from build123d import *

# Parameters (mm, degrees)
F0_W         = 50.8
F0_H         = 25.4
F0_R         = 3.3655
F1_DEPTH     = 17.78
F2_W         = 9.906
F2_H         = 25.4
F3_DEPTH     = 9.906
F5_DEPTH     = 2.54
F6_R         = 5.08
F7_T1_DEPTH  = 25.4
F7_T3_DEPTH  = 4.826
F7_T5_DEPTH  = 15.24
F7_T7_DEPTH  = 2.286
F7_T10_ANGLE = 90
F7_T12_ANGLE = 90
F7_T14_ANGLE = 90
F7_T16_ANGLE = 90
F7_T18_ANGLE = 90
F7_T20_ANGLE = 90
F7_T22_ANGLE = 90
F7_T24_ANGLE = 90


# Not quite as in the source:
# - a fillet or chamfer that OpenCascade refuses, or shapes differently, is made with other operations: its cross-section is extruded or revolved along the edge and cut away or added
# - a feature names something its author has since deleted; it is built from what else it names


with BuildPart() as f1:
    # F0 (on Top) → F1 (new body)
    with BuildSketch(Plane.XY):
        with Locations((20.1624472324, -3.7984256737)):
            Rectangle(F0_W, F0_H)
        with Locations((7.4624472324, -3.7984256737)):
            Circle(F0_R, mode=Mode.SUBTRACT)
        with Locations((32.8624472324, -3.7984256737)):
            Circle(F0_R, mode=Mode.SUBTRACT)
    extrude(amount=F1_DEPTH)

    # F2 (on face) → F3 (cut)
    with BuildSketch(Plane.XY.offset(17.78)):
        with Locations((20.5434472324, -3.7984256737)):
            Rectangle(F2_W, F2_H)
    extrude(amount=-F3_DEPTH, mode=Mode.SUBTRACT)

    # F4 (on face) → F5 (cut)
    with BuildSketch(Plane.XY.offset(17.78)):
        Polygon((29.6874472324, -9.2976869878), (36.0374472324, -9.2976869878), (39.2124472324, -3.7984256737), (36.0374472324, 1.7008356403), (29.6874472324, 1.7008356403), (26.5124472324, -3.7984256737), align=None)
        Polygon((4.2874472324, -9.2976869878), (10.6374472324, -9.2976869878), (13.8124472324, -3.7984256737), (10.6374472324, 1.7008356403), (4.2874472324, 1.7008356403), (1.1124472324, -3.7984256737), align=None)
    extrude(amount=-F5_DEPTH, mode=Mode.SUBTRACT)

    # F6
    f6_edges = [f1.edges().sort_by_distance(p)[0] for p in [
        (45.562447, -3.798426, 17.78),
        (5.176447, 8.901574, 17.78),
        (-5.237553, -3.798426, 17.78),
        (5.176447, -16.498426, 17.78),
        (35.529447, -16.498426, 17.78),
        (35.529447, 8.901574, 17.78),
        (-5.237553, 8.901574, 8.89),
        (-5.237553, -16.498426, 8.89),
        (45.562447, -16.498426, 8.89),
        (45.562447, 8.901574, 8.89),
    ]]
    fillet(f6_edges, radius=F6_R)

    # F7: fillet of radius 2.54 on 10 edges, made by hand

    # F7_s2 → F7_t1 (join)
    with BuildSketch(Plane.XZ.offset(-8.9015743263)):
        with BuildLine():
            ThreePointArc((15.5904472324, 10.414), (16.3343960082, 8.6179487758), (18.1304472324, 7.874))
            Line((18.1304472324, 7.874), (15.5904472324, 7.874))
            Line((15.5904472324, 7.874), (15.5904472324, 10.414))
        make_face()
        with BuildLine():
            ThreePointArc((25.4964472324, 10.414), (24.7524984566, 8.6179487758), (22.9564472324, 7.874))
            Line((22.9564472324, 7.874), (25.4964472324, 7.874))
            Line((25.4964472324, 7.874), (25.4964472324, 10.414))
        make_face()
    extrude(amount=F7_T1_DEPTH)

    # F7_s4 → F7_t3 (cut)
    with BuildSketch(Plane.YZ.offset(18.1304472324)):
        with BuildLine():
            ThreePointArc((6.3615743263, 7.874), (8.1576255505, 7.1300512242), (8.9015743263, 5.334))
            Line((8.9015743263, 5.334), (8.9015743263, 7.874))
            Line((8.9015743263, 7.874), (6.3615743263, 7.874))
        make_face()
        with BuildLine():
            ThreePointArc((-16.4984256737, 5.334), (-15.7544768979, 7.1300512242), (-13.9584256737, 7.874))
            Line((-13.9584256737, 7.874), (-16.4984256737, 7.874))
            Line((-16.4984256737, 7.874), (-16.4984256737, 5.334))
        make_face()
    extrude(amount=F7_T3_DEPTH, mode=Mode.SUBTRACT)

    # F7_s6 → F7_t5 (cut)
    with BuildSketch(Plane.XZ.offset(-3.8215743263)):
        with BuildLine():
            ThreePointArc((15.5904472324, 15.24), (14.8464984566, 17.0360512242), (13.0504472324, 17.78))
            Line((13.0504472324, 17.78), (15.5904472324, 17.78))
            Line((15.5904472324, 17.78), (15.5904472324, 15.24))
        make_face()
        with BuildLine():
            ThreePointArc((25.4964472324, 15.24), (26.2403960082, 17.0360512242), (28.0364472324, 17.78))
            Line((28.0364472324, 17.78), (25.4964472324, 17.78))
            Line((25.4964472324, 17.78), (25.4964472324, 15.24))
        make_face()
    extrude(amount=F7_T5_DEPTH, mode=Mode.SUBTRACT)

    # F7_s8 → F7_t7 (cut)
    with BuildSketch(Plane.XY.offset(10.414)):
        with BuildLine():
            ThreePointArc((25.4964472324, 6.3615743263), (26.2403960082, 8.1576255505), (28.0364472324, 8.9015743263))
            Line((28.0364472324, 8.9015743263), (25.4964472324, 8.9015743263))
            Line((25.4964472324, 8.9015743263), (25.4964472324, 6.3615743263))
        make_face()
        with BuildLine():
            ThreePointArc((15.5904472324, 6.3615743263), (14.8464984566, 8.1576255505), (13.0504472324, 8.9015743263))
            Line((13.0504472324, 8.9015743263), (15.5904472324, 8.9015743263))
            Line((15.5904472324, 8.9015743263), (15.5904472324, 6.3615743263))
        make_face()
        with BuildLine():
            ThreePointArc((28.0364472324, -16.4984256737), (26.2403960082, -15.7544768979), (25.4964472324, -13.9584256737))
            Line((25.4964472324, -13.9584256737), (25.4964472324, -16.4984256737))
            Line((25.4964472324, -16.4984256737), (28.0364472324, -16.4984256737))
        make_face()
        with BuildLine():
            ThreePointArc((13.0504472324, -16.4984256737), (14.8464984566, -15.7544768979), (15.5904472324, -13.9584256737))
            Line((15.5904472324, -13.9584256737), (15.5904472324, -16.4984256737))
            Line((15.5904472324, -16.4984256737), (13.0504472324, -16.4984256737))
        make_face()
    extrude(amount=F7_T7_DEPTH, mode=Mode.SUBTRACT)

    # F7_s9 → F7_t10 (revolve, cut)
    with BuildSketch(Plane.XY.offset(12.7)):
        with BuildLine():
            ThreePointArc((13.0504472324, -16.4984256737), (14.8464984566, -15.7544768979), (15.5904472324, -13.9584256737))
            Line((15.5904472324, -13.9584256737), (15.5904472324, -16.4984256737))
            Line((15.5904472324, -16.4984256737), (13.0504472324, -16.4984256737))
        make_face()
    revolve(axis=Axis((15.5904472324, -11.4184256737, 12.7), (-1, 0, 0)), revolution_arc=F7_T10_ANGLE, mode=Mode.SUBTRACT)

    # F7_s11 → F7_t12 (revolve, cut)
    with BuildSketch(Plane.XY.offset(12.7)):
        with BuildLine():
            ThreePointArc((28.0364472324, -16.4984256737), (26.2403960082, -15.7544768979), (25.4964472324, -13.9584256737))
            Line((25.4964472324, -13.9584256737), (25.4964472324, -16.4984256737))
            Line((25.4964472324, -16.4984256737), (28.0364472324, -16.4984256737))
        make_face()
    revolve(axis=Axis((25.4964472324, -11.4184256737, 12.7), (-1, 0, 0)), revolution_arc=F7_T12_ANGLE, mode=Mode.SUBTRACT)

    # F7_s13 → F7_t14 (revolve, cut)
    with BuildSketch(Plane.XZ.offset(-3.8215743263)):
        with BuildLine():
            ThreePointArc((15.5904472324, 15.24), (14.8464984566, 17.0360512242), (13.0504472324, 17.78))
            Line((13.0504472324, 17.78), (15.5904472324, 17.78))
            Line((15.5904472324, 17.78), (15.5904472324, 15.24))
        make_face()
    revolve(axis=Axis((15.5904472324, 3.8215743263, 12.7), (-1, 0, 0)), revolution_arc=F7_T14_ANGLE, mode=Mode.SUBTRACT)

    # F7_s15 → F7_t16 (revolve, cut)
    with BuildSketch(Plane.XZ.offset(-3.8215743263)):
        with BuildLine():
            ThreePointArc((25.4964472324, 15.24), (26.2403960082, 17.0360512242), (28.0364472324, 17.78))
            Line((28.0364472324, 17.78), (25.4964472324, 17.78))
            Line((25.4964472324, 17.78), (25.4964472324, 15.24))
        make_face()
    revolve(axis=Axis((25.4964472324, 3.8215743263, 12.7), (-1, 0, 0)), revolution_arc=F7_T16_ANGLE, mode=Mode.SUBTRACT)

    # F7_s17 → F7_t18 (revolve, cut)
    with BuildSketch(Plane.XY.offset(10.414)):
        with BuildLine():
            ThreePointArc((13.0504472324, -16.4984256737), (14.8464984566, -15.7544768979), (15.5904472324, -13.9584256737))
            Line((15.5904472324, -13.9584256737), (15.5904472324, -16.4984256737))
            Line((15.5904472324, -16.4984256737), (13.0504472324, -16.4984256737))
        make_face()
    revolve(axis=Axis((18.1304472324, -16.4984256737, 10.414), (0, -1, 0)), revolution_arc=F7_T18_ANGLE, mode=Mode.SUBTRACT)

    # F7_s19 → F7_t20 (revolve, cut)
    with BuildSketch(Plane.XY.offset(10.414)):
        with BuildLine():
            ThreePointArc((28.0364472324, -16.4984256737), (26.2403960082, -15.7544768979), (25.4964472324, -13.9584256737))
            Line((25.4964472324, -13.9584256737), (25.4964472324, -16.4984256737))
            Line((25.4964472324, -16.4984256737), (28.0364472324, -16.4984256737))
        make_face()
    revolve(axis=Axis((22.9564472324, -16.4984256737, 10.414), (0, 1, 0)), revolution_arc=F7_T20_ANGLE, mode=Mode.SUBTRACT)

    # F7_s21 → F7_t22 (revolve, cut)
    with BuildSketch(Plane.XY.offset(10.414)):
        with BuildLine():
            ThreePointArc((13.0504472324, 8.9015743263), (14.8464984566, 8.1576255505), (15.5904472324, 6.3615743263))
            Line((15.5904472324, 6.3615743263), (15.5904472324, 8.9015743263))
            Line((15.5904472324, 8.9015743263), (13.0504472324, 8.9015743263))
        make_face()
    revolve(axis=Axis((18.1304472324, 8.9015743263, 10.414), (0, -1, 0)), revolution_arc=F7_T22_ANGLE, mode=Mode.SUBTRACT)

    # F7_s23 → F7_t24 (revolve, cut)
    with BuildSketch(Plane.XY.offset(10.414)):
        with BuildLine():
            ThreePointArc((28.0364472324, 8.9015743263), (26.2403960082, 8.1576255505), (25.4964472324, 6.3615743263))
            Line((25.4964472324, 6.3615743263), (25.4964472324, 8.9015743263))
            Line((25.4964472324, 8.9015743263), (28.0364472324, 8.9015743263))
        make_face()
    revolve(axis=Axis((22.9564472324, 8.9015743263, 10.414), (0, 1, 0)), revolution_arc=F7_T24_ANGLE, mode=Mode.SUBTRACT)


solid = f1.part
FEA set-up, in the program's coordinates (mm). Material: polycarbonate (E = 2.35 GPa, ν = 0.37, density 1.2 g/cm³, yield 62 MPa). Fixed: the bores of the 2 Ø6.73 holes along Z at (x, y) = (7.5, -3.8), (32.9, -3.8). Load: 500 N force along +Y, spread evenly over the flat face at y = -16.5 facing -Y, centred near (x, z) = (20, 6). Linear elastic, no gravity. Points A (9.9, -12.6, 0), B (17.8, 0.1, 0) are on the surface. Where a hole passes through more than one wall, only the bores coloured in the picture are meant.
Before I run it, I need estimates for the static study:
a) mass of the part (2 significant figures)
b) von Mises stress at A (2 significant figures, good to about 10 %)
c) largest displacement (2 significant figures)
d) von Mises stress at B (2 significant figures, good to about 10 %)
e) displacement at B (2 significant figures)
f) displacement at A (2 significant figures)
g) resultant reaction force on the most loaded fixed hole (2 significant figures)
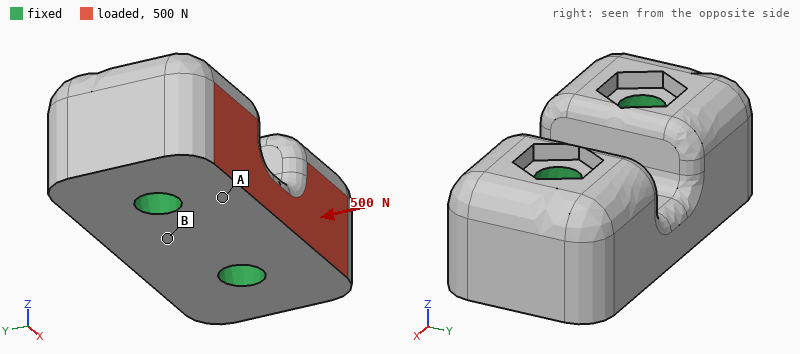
21 g
1.4 MPa
10 µm
0.41 MPa
2.9 µm
5.5 µm
250 N
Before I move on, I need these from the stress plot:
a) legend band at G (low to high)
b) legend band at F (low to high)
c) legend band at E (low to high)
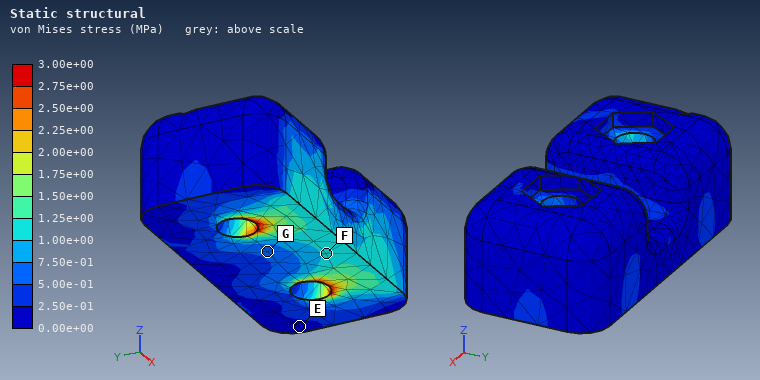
5.00e-01 to 7.50e-01 MPa
1.00e+00 to 1.25e+00 MPa
0.00e+00 to 2.50e-01 MPa
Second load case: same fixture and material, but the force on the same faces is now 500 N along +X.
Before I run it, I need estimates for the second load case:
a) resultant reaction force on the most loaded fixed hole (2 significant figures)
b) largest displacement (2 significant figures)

290 N
21 µm
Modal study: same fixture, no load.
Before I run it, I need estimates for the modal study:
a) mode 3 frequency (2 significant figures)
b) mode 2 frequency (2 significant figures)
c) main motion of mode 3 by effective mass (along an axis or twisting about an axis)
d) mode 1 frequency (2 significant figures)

11 kHz
9900 Hz
twisting about X
9600 Hz
